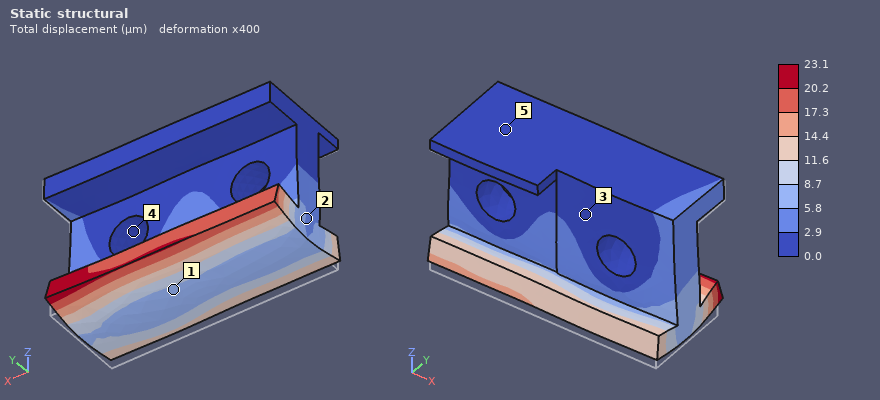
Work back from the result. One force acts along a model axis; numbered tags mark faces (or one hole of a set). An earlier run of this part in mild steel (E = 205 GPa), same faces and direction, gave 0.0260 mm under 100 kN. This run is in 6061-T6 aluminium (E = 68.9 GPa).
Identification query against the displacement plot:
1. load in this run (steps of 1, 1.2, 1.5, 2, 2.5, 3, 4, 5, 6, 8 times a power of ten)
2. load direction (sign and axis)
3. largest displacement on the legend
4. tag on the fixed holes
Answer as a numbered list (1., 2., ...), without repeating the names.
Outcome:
1. 30 kN
2. +Z
3. 23.1 µm
4. 4
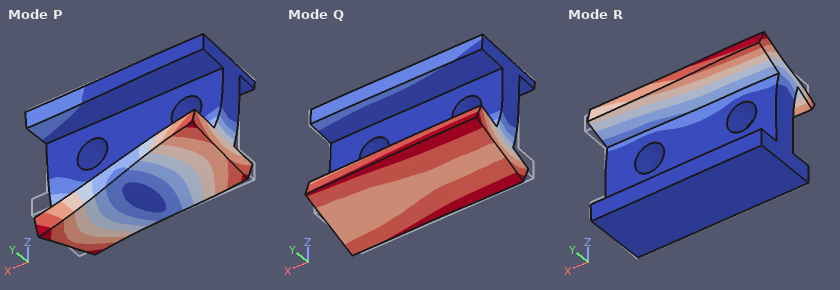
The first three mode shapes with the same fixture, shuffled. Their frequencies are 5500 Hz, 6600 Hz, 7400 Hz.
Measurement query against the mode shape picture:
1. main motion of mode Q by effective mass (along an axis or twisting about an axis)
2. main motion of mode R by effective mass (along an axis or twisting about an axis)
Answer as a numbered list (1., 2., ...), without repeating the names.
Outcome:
1. along Y
2. along Y
